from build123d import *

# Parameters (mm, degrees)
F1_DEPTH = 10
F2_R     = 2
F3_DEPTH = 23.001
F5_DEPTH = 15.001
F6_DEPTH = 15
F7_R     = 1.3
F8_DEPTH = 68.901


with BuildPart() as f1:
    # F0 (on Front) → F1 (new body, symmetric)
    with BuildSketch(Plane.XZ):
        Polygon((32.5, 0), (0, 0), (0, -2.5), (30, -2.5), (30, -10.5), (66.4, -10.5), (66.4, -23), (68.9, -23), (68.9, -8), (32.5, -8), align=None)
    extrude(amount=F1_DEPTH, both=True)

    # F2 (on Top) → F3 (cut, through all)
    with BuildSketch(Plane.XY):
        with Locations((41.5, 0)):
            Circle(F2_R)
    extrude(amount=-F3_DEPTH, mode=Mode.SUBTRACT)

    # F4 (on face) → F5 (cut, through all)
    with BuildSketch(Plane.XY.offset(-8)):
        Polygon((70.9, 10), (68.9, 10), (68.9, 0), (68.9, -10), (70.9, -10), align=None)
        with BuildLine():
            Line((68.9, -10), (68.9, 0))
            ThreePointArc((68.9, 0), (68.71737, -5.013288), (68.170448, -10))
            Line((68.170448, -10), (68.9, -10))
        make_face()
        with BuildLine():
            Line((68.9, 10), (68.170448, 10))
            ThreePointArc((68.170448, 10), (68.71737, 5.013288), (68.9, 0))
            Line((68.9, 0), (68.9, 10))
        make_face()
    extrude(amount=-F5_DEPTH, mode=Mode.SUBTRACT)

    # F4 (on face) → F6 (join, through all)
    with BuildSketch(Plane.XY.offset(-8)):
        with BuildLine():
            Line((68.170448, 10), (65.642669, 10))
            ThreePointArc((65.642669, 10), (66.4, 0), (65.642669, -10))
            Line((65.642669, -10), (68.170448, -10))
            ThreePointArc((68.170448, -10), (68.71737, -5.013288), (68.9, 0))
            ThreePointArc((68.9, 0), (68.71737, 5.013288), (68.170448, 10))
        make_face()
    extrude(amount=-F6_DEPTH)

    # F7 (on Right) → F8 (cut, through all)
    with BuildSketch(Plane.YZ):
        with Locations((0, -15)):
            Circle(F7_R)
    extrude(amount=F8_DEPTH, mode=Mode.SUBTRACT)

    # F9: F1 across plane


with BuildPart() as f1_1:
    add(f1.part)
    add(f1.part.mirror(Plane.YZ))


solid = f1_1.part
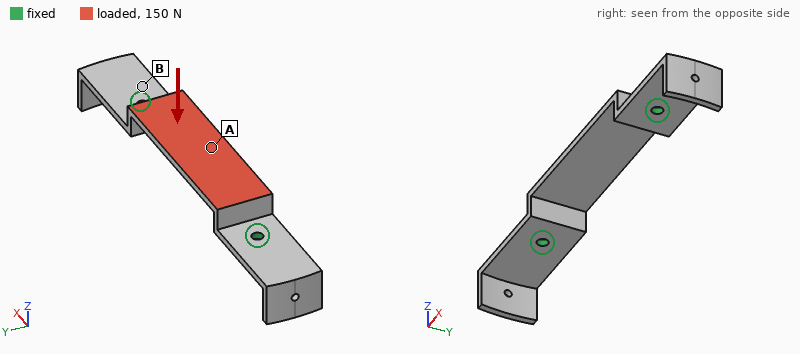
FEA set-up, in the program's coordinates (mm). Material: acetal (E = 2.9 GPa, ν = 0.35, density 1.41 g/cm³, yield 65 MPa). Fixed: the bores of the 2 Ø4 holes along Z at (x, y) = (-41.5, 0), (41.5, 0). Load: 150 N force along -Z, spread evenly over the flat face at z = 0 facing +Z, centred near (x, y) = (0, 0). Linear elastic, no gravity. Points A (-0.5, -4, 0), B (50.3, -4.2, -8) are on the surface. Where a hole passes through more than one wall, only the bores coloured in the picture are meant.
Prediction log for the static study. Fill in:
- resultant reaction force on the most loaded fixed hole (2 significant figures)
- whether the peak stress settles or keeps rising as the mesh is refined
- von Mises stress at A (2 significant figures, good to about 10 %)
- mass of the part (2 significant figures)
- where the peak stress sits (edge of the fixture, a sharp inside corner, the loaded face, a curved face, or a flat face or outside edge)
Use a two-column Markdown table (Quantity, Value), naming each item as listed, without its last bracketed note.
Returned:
| Quantity | Value |
|---|---|
| resultant reaction force on the most loaded fixed hole | 160 N |
| whether the peak stress settles or keeps rising as the mesh is refined | keeps rising |
| von Mises stress at A | 21 MPa |
| mass of the part | 12 g |
| where the peak stress sits | edge of the fixture |
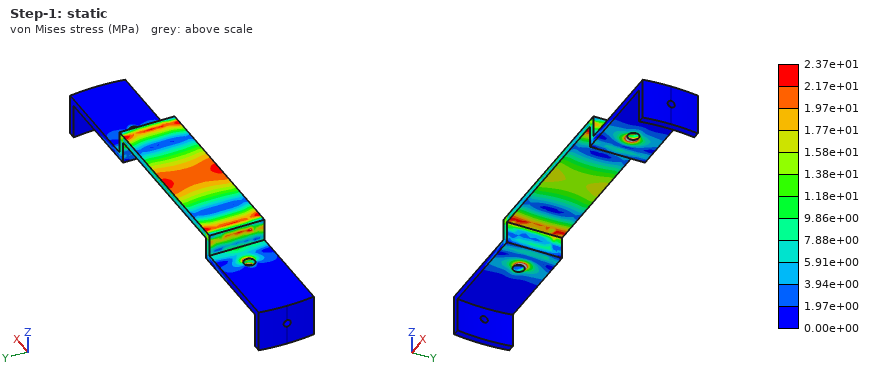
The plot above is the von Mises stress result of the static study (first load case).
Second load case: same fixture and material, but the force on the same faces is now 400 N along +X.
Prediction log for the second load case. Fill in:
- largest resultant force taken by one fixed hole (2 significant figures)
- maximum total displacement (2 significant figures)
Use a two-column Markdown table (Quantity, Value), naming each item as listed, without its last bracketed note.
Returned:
| Quantity | Value |
|---|---|
| largest resultant force taken by one fixed hole | 200 N |
| maximum total displacement | 1.2 mm |
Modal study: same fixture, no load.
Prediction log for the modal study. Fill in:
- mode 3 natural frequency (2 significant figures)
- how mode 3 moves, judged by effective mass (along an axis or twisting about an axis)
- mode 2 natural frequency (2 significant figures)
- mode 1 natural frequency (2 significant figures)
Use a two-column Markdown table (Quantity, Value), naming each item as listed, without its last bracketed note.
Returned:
| Quantity | Value |
|---|---|
| mode 3 natural frequency | 850 Hz |
| how mode 3 moves, judged by effective mass | along Z |
| mode 2 natural frequency | 470 Hz |
| mode 1 natural frequency | 470 Hz |
